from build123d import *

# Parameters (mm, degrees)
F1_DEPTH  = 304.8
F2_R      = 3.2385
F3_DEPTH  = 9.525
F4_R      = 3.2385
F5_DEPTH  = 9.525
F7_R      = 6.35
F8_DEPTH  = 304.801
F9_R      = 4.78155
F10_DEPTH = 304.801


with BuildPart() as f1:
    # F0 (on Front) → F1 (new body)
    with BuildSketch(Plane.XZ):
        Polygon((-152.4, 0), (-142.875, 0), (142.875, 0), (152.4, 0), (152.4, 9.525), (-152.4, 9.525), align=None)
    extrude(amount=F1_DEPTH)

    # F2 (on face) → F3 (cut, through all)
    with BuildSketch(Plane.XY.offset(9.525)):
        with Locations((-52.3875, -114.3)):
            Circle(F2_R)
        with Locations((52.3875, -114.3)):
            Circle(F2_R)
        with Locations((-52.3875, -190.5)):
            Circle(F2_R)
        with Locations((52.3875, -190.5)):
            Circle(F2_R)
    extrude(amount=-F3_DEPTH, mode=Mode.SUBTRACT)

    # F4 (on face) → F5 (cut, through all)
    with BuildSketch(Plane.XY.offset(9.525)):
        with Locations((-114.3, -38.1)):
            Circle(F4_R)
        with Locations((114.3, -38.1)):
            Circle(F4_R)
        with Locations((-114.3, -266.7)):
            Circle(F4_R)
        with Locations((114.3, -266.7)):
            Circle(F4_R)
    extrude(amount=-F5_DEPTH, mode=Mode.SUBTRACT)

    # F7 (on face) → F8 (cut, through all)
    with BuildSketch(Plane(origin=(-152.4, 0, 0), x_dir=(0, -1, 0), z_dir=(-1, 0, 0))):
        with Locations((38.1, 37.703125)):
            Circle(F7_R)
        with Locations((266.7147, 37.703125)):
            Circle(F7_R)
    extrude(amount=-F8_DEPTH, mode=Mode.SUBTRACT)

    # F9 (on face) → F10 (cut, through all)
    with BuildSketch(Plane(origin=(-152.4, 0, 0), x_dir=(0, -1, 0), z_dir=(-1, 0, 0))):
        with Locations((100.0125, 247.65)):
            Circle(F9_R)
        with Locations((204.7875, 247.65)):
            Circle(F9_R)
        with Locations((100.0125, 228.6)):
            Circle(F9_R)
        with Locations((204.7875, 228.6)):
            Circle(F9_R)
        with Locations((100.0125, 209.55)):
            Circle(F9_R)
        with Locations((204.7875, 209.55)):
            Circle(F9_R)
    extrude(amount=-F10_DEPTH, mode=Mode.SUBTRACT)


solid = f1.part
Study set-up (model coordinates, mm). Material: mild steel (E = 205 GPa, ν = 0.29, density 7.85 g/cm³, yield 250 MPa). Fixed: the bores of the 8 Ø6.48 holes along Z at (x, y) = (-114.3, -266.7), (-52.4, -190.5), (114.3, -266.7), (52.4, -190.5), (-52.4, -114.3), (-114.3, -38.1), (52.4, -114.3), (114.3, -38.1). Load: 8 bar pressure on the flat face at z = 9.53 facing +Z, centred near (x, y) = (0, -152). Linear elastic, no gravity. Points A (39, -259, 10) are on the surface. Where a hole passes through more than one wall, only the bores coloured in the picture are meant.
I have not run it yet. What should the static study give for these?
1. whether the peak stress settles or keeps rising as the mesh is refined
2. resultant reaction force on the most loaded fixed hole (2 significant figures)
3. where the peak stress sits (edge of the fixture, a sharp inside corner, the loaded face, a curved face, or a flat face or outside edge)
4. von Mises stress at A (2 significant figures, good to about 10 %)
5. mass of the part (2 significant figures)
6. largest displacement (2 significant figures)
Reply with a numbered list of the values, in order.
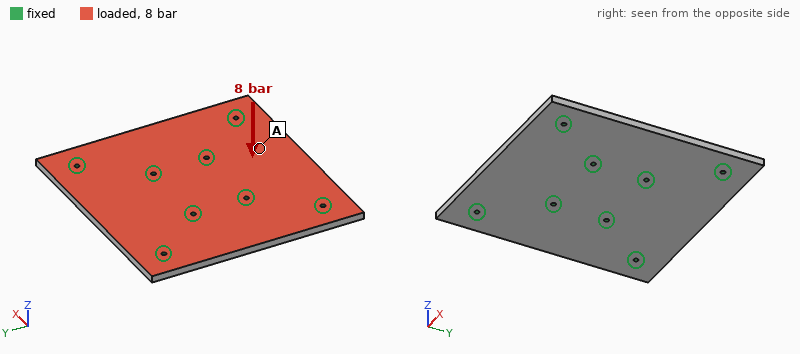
1. keeps rising
2. 9.3 kN
3. edge of the fixture
4. 43 MPa
5. 6.9 kg
6. 0.33 mm
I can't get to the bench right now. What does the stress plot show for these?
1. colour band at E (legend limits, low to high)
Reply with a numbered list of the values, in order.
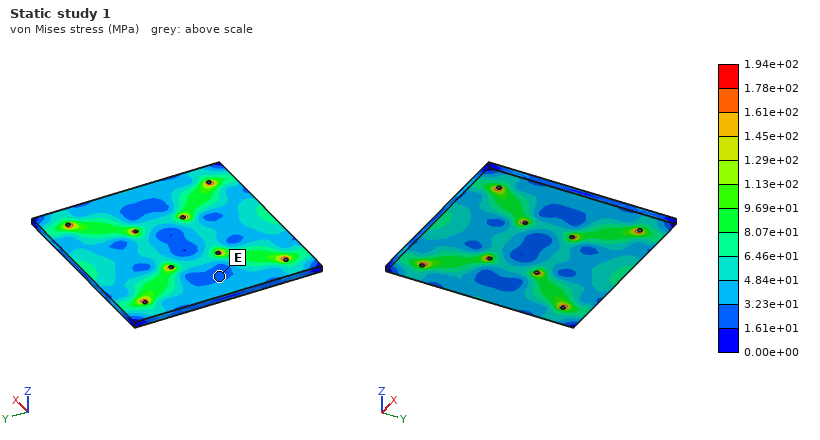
1. 1.61e+01 to 3.23e+01 MPa
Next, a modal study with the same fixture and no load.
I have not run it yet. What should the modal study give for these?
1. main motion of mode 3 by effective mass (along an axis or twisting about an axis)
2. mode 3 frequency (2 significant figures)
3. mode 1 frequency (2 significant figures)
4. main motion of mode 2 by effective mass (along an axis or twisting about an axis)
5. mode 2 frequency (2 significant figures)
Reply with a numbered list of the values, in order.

1. twisting about Y
2. 1300 Hz
3. 1000 Hz
4. twisting about X
5. 1100 Hz
